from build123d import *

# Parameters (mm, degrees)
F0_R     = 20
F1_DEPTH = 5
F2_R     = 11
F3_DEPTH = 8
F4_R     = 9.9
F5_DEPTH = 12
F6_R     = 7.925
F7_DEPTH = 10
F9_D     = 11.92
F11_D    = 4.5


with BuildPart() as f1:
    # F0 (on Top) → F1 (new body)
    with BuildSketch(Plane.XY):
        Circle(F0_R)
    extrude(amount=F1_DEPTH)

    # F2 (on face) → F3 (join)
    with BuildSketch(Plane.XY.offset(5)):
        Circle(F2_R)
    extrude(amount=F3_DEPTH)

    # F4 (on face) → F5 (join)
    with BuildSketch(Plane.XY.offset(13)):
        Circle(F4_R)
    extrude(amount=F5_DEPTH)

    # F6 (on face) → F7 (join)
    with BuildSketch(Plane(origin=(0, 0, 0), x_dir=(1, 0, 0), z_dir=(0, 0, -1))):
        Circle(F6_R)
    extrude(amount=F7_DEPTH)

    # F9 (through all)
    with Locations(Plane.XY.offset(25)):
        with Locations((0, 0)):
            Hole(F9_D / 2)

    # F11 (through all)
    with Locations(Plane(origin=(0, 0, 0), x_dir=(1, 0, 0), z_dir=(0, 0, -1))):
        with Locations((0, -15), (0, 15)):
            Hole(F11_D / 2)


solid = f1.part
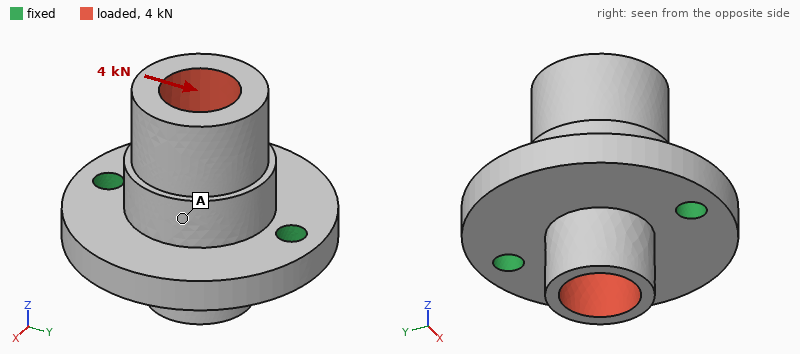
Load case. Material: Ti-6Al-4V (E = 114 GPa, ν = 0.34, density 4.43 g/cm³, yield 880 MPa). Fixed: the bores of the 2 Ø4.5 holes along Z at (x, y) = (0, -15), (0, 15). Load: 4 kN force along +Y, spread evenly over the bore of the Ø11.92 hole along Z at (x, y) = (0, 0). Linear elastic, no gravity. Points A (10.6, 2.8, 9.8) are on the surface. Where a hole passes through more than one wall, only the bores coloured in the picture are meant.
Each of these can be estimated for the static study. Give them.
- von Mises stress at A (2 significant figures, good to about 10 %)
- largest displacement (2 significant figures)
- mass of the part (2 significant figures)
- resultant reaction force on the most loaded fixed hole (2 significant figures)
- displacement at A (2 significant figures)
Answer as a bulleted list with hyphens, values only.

- 12 MPa
- 11 µm
- 48 g
- 2.1 kN
- 4.3 µm
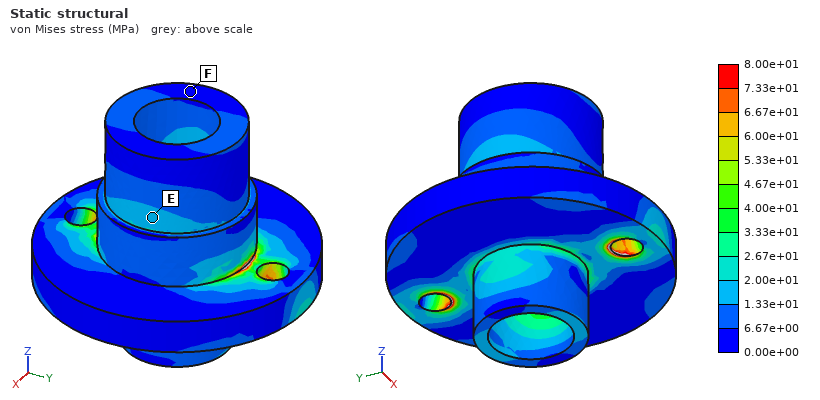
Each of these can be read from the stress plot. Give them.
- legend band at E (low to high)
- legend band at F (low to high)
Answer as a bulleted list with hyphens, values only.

- 1.33e+01 to 2.00e+01 MPa
- 0.00e+00 to 6.67e+00 MPa
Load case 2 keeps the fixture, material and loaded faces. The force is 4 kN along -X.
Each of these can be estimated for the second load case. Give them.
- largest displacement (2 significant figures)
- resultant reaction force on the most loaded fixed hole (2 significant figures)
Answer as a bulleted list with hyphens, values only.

- 49 µm
- 2.0 kN
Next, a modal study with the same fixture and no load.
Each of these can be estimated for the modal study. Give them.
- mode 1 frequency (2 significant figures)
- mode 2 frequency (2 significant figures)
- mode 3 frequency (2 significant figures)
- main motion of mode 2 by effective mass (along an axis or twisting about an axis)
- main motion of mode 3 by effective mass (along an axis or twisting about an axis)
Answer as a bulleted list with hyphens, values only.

- 6500 Hz
- 16 kHz
- 18 kHz
- along Z
- along Y
